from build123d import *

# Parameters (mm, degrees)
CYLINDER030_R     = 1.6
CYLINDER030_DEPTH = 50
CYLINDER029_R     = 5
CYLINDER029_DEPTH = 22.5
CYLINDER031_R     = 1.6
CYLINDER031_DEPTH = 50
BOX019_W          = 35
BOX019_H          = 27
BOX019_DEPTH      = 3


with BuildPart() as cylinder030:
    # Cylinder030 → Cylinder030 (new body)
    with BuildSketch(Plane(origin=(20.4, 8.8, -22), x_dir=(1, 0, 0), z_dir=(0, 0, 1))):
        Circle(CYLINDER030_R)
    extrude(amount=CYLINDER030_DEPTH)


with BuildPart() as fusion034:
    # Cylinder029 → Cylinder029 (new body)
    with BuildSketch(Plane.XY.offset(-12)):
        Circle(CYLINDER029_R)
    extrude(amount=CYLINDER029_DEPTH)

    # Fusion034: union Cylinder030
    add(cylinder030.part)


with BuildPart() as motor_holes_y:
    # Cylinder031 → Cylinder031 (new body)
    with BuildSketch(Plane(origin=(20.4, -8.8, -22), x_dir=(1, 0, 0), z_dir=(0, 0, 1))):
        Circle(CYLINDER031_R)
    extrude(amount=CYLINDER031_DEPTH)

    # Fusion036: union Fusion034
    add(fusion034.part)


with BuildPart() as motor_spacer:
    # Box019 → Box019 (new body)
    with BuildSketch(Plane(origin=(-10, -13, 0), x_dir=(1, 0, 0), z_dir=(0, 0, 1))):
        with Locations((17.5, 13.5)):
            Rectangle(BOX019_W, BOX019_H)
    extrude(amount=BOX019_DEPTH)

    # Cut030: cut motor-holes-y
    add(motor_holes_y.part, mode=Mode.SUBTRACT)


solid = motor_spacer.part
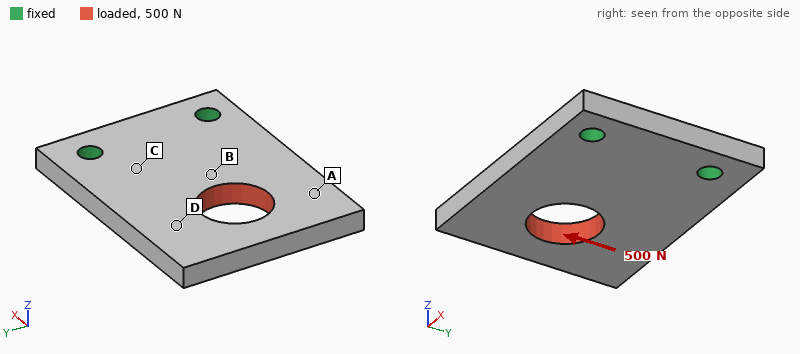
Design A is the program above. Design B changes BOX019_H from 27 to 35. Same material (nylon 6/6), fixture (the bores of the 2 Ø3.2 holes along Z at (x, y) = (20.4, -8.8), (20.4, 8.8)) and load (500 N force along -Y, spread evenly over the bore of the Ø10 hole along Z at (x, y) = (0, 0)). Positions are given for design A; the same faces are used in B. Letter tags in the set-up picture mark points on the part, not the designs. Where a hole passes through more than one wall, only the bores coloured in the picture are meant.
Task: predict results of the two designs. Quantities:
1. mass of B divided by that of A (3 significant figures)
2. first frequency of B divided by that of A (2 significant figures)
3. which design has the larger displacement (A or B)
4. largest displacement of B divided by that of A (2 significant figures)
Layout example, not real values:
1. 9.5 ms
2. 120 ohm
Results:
1. 1.33
2. 0.98
3. A
4. 0.85
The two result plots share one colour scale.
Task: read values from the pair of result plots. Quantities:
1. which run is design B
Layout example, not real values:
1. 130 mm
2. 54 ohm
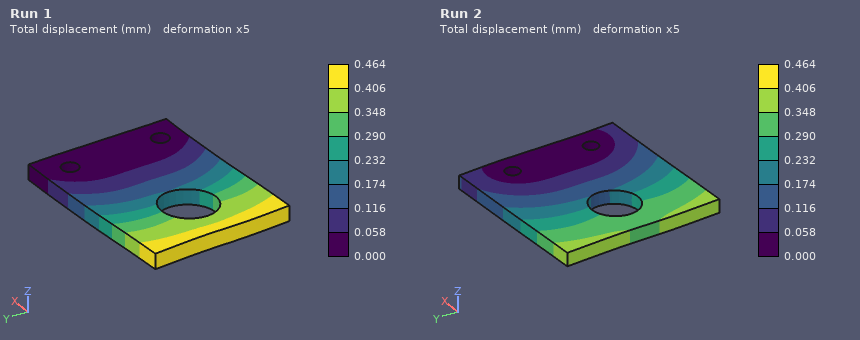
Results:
1. Run 2
